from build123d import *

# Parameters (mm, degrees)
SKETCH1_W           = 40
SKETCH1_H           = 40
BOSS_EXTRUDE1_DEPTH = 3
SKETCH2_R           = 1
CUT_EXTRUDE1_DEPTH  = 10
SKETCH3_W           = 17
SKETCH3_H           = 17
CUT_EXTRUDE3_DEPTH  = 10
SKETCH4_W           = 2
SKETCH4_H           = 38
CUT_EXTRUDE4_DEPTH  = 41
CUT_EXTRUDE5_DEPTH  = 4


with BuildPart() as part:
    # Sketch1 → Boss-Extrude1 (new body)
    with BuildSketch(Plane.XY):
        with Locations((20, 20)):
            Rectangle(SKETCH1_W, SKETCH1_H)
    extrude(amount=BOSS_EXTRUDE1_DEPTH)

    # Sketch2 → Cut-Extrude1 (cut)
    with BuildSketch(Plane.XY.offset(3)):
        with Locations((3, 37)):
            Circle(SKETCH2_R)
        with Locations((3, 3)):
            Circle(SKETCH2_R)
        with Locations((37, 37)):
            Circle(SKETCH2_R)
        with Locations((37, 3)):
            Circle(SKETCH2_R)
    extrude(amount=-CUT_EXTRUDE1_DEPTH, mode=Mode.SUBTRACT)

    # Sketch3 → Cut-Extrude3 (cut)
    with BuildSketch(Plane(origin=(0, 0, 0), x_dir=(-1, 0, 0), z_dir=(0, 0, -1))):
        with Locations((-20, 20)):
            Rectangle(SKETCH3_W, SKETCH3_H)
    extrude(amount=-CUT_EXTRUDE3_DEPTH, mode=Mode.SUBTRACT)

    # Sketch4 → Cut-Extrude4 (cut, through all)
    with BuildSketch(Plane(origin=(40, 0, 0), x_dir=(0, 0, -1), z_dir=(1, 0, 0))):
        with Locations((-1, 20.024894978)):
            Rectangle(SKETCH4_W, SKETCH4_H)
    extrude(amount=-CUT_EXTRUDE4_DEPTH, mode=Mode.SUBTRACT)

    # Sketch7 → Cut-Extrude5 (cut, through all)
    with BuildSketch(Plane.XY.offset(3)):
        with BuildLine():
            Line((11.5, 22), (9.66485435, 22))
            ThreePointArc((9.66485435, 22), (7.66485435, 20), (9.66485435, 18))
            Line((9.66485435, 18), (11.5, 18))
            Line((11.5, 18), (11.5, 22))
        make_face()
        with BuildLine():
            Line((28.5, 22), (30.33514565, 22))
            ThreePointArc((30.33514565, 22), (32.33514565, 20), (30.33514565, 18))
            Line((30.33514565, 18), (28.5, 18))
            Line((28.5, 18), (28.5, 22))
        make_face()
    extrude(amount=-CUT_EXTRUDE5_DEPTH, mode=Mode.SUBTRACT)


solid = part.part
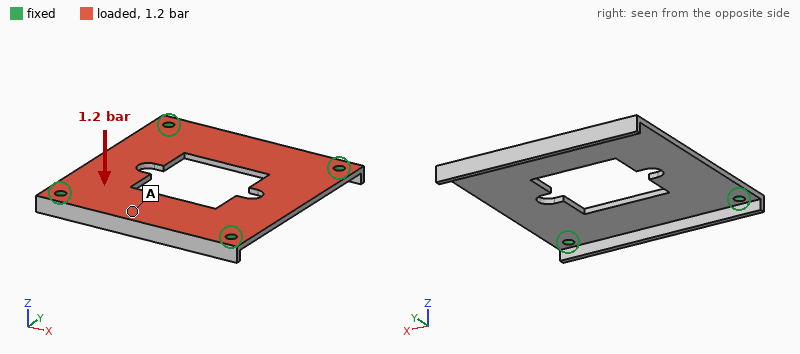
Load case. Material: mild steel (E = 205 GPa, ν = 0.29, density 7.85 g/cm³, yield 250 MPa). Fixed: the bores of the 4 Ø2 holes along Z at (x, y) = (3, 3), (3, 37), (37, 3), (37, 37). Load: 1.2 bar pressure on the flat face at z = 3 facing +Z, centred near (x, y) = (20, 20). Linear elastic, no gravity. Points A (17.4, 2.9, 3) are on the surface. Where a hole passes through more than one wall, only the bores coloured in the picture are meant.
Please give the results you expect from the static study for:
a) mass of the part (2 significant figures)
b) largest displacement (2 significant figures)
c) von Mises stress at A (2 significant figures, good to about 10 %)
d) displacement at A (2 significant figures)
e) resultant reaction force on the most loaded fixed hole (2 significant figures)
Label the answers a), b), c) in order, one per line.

a) 11 g
b) 45 µm
c) 17 MPa
d) 11 µm
e) 40 N
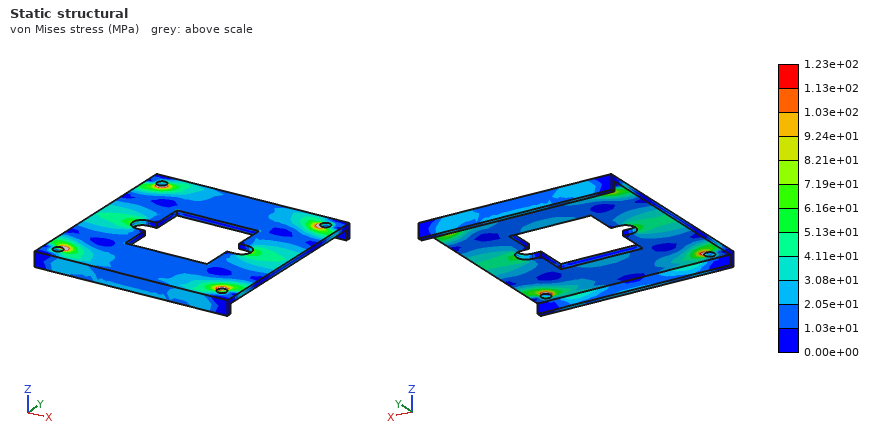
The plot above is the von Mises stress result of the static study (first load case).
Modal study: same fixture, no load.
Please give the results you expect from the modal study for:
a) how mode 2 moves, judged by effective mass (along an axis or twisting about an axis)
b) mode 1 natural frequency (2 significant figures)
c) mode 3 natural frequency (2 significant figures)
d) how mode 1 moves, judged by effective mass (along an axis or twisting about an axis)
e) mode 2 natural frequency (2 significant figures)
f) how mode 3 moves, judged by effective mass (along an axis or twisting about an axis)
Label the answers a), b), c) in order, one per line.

a) twisting about Y
b) 3900 Hz
c) 6200 Hz
d) along Z
e) 5000 Hz
f) twisting about X
